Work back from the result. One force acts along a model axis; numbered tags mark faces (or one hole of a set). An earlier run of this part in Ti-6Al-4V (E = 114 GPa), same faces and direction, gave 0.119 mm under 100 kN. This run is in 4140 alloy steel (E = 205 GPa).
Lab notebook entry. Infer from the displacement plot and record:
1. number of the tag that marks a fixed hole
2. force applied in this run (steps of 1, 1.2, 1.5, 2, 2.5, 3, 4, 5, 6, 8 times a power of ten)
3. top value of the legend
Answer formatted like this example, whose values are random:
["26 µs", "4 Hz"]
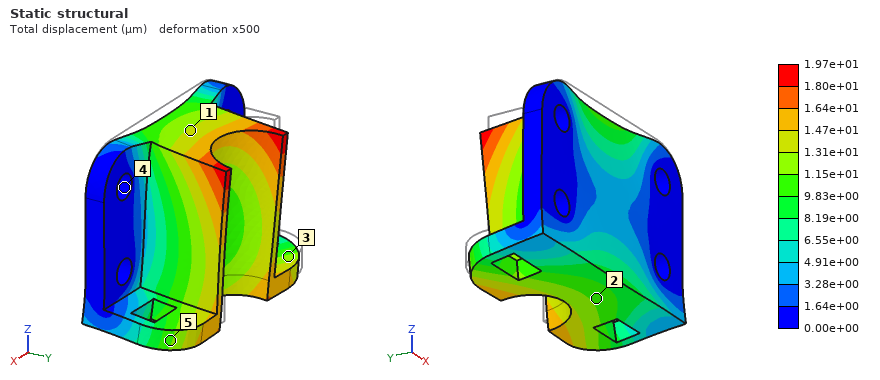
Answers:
["4", "30 kN", "1.97e+01 µm"]
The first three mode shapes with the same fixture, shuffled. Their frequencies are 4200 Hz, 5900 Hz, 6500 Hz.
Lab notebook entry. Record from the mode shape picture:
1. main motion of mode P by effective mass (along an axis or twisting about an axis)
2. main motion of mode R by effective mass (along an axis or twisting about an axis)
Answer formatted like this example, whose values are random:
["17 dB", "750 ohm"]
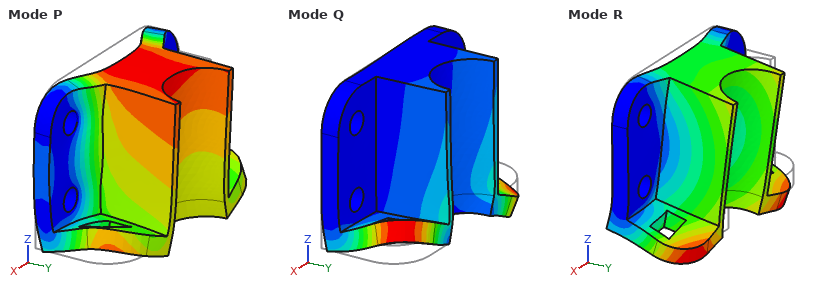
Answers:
["along Y", "along Z"]
